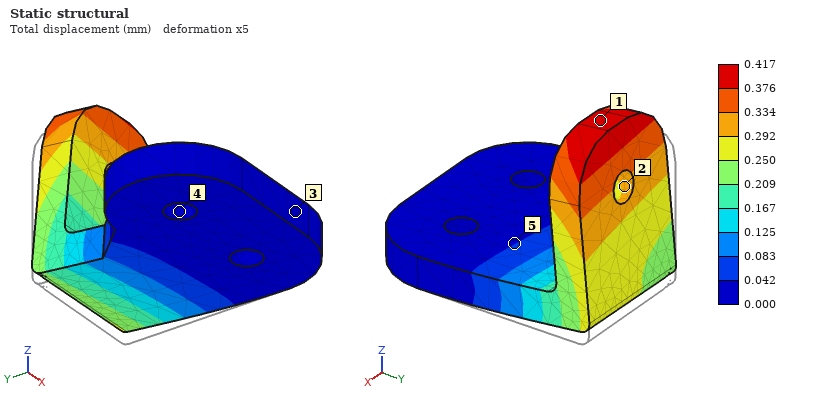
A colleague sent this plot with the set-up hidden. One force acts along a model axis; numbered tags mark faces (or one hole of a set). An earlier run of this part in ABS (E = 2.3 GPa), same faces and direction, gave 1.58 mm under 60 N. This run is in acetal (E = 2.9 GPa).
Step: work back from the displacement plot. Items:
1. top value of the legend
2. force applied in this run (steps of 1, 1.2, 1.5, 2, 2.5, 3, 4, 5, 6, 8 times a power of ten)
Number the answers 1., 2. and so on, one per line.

1. 0.417 mm
2. 20 N
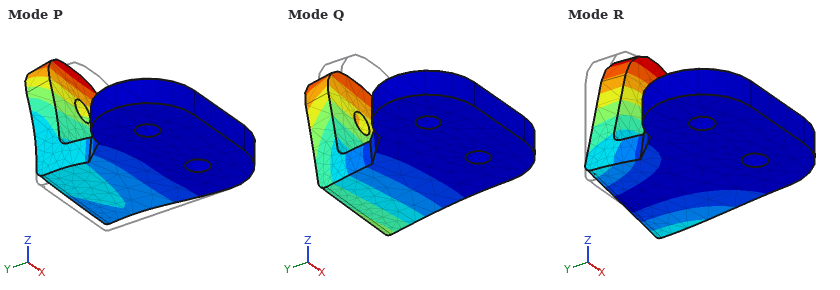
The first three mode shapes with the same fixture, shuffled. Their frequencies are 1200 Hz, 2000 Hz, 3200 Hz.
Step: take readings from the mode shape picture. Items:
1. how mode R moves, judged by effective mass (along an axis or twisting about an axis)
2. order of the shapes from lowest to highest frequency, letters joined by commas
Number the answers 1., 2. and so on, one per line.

1. along X
2. Q, R, P
